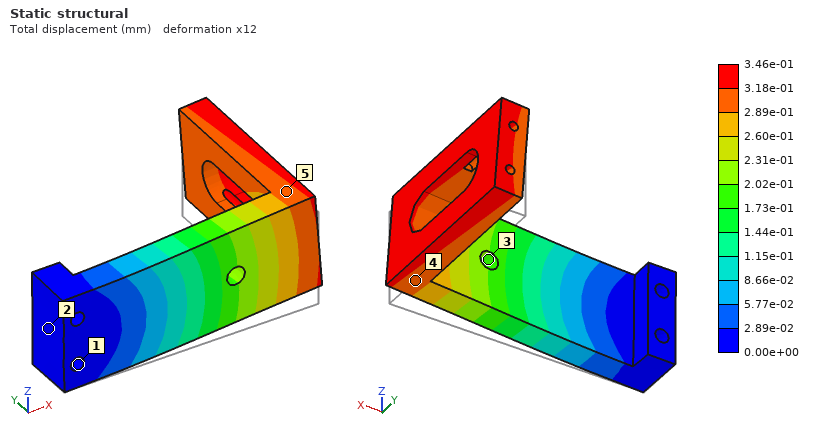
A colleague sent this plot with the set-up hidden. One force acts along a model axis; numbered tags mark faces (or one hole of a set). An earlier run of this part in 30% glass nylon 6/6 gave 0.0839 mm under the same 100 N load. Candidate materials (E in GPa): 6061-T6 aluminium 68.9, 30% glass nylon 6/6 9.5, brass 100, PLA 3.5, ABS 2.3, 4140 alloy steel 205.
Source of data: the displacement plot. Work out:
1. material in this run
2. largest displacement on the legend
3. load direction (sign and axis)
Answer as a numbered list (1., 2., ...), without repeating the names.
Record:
1. ABS
2. 3.46e-01 mm
3. +Z
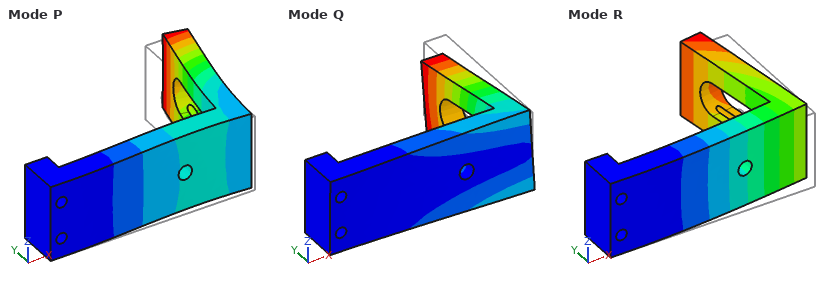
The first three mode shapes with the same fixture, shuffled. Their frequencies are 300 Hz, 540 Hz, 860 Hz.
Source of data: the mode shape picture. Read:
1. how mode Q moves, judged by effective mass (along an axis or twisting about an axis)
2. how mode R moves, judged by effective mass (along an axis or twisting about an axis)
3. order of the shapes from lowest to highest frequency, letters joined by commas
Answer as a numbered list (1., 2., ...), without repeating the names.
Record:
1. along Z
2. along Y
3. R, Q, P
